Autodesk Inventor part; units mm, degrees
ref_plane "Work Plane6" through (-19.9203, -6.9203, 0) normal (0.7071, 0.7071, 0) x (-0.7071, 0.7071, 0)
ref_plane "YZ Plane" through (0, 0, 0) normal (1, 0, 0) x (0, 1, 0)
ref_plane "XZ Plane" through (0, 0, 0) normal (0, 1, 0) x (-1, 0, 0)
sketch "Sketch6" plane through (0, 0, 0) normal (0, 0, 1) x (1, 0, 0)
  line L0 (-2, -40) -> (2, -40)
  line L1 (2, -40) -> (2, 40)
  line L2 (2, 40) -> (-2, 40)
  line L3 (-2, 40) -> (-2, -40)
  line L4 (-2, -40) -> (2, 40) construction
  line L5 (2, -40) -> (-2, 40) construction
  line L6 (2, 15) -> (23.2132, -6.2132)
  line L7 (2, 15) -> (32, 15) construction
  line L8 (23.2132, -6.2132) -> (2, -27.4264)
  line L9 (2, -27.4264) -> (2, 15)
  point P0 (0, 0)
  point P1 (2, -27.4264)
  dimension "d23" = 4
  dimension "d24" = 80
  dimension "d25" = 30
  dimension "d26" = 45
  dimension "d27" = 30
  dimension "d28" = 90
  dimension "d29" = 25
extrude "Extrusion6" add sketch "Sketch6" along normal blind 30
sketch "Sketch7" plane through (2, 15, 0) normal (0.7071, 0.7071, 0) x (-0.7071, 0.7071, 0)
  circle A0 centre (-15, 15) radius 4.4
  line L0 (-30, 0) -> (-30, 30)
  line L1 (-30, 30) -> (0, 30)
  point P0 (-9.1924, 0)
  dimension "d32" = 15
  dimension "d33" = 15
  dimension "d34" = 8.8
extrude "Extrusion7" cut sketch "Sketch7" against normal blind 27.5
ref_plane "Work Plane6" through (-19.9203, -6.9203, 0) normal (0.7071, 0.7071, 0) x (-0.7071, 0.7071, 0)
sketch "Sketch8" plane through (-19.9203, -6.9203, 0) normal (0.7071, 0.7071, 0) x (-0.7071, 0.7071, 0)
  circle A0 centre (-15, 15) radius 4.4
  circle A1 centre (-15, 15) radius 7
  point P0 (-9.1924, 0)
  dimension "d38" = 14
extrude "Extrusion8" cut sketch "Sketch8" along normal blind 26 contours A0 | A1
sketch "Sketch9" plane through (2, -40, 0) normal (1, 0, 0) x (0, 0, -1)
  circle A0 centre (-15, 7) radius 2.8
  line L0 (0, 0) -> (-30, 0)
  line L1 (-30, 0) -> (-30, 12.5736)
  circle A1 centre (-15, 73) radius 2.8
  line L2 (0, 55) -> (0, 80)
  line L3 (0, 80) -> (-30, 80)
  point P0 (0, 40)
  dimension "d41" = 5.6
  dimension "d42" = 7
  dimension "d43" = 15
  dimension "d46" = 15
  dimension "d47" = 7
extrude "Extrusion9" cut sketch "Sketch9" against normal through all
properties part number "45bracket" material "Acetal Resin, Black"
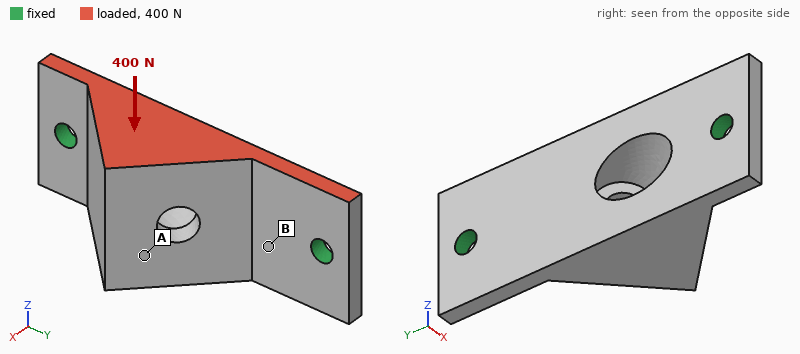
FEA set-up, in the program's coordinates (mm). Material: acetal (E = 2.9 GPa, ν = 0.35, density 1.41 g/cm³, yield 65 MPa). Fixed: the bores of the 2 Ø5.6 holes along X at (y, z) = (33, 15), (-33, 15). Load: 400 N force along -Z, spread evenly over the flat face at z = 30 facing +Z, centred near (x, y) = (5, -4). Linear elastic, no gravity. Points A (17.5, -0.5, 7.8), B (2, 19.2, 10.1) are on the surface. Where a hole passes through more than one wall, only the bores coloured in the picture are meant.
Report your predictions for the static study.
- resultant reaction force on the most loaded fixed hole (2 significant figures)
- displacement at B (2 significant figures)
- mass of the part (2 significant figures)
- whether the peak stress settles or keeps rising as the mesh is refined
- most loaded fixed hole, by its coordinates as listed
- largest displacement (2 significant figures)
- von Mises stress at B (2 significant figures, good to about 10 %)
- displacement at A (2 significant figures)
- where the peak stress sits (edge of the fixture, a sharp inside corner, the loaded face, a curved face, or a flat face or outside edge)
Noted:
230 N
0.076 mm
28 g
keeps rising
(-33, 15)
0.45 mm
6.4 MPa
0.32 mm
edge of the fixture
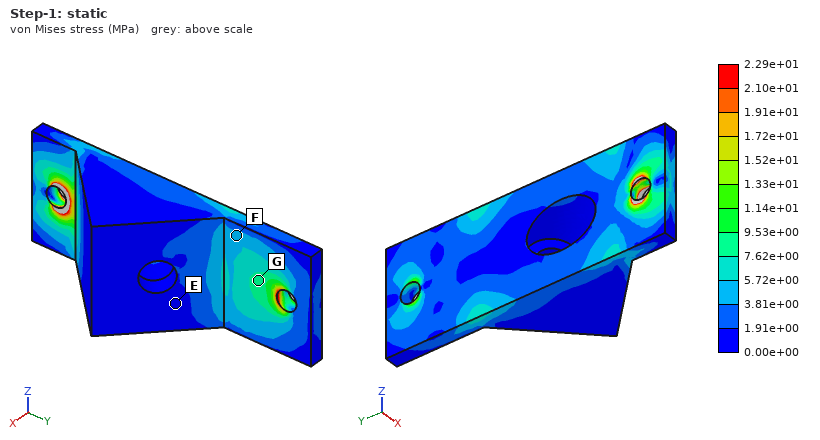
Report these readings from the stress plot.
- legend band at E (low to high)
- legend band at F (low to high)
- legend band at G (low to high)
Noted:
0.00e+00 to 1.91e+00 MPa
3.81e+00 to 5.72e+00 MPa
7.62e+00 to 9.53e+00 MPa
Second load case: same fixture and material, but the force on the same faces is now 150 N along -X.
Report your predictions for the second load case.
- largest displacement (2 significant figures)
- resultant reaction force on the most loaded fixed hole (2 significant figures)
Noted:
0.42 mm
100 N
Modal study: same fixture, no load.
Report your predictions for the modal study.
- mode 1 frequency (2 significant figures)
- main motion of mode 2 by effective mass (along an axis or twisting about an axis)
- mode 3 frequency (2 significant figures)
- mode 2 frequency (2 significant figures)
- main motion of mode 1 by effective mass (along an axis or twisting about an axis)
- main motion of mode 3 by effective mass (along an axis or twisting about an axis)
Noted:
960 Hz
along X
3300 Hz
1400 Hz
along Z
along Z
